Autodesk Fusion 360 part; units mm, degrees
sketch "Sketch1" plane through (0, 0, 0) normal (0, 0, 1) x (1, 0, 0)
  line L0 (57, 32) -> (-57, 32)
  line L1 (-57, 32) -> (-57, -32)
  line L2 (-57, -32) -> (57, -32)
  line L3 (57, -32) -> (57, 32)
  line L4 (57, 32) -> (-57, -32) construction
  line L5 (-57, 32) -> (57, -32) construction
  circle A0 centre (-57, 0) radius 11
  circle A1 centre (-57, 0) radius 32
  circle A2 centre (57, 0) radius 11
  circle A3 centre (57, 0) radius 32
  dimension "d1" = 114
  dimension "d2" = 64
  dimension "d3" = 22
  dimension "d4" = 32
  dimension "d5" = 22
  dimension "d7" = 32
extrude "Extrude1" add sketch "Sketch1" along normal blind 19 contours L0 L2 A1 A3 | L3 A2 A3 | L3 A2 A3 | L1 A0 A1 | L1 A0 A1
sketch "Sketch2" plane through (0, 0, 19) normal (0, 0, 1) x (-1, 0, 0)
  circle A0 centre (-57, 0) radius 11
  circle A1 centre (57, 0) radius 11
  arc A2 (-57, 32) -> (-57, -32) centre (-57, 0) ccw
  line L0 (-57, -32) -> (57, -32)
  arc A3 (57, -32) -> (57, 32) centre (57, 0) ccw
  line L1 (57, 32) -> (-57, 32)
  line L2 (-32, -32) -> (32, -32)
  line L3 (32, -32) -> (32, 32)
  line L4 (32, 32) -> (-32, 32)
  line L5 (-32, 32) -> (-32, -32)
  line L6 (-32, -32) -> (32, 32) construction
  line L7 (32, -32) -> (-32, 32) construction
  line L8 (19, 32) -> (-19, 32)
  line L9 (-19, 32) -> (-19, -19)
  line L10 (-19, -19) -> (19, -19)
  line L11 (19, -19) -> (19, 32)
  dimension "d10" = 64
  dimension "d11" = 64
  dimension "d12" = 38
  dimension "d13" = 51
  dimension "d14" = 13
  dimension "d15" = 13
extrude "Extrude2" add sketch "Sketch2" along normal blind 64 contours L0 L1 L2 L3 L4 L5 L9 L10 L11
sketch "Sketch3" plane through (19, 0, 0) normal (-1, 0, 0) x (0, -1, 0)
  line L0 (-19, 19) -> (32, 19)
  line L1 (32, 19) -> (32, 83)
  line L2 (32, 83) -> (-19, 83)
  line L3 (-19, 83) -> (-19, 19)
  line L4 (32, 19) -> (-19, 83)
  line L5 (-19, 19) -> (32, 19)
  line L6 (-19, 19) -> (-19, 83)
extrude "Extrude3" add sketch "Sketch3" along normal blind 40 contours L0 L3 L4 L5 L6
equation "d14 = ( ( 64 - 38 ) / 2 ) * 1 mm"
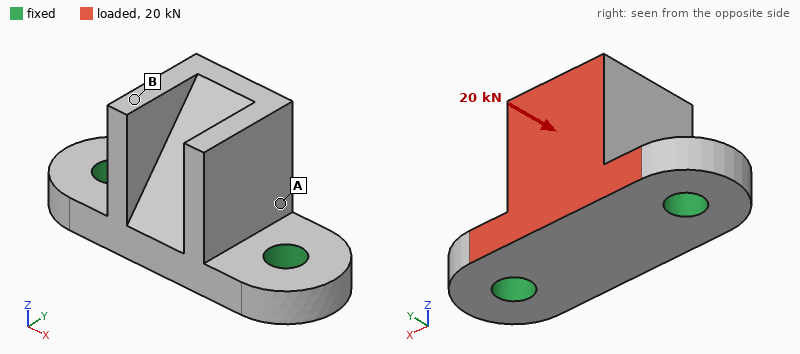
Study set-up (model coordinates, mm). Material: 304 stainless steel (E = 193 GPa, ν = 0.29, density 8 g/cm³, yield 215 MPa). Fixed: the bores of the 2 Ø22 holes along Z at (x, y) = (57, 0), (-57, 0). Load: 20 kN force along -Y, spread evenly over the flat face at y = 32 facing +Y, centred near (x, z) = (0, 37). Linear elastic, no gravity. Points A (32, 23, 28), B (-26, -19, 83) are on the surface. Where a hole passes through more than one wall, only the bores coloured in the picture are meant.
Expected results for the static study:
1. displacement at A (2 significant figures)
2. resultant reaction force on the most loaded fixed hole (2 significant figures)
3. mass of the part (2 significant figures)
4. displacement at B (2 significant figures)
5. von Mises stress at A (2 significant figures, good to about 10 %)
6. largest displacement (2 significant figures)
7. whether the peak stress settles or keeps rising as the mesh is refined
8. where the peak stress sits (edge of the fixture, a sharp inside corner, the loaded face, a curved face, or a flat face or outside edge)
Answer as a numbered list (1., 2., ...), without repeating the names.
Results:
1. 20 µm
2. 10 kN
3. 3.1 kg
4. 51 µm
5. 21 MPa
6. 55 µm
7. keeps rising
8. edge of the fixture
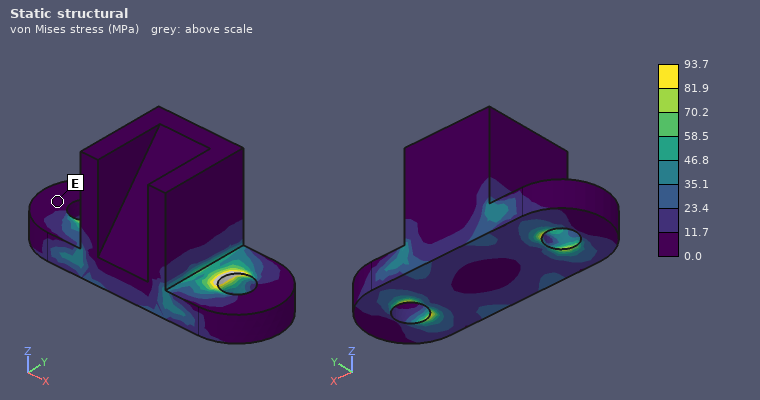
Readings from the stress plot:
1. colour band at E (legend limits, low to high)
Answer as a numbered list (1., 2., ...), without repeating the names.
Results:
1. 0.0 to 11.7 MPa
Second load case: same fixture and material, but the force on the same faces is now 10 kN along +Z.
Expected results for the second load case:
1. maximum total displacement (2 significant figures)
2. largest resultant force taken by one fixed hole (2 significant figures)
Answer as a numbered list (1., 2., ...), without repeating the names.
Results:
1. 28 µm
2. 5.3 kN
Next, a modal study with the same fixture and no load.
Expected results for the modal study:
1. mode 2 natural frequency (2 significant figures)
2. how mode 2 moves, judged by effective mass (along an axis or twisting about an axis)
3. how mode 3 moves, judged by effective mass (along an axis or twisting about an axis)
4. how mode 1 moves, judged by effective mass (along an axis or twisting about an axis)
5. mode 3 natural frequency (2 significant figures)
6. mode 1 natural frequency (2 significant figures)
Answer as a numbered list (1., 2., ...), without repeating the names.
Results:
1. 4700 Hz
2. along X
3. along Z
4. along Y
5. 5500 Hz
6. 2400 Hz
